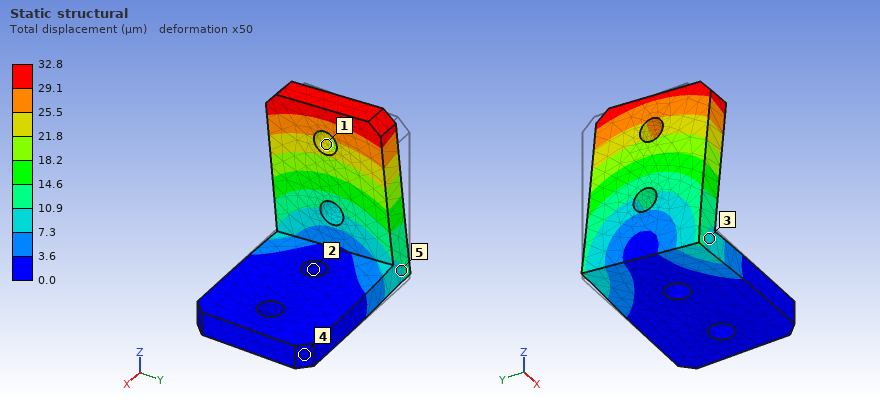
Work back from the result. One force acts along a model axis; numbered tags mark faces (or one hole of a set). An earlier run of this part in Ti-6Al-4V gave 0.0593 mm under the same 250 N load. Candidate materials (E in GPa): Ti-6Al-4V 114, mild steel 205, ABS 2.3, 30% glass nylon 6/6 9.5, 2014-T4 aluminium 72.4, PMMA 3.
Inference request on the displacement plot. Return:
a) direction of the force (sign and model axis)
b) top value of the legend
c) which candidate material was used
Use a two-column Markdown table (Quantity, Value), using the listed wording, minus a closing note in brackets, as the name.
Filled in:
| Quantity | Value |
|---|---|
| direction of the force | -Y |
| top value of the legend | 32.8 µm |
| which candidate material was used | mild steel |
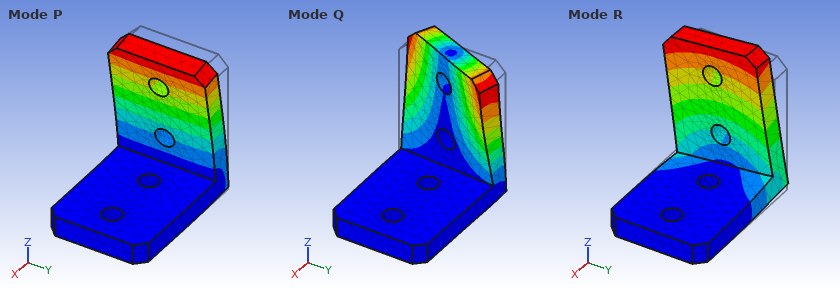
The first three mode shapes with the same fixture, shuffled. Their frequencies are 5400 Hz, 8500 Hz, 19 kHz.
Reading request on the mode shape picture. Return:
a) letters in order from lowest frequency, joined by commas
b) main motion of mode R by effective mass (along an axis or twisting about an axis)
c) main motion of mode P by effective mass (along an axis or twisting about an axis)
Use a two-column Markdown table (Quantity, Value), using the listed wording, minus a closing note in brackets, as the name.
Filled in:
| Quantity | Value |
|---|---|
| letters in order from lowest frequency, joined by commas | P, R, Q |
| main motion of mode R by effective mass | along Y |
| main motion of mode P by effective mass | along X |
